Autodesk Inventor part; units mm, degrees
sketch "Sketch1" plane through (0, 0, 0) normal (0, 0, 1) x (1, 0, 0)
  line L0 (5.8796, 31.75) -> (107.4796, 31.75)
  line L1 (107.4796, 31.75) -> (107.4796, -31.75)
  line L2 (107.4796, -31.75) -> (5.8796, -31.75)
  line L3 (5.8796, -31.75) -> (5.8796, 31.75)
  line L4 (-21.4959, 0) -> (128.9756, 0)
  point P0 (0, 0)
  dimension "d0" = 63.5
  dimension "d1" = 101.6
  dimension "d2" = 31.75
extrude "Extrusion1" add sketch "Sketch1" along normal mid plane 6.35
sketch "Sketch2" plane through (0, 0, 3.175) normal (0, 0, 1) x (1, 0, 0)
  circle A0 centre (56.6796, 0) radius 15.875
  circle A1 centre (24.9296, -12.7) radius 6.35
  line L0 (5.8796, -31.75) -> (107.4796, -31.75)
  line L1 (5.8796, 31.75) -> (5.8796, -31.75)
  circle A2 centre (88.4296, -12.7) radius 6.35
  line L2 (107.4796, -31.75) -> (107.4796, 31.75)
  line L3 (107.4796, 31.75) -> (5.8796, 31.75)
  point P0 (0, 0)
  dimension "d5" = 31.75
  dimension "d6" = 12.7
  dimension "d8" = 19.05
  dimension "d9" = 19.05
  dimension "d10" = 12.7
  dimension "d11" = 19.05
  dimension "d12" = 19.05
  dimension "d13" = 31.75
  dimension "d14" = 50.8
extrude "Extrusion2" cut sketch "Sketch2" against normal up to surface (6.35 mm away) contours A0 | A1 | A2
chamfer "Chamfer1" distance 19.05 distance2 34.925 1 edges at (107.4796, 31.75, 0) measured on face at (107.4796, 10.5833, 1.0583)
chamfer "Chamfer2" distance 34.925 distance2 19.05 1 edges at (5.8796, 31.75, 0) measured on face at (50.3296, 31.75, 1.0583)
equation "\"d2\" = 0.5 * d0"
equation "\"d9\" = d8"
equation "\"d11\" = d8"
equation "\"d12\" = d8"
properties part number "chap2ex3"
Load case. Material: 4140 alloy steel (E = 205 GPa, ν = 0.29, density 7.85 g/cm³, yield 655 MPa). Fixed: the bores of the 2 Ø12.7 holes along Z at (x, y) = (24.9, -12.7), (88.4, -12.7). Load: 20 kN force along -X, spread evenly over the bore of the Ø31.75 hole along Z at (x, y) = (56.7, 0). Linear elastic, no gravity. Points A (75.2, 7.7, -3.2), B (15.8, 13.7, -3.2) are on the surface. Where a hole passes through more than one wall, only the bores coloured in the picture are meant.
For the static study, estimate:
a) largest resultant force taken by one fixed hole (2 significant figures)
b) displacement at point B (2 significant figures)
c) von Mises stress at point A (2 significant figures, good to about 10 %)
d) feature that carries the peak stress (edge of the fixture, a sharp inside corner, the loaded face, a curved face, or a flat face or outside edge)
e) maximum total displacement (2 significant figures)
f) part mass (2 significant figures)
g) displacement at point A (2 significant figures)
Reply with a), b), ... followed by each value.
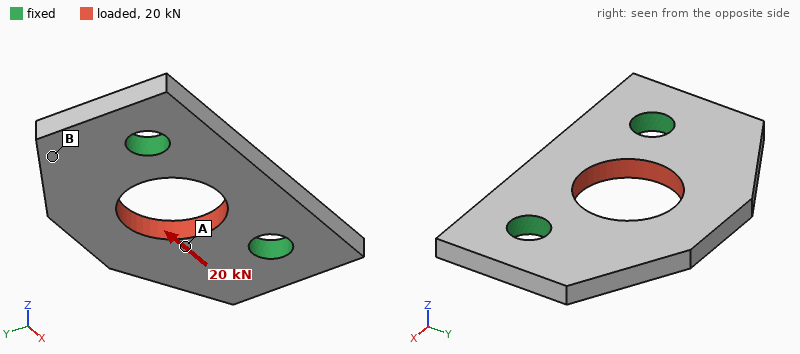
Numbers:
a) 10 kN
b) 12 µm
c) 61 MPa
d) edge of the fixture
e) 19 µm
f) 240 g
g) 13 µm
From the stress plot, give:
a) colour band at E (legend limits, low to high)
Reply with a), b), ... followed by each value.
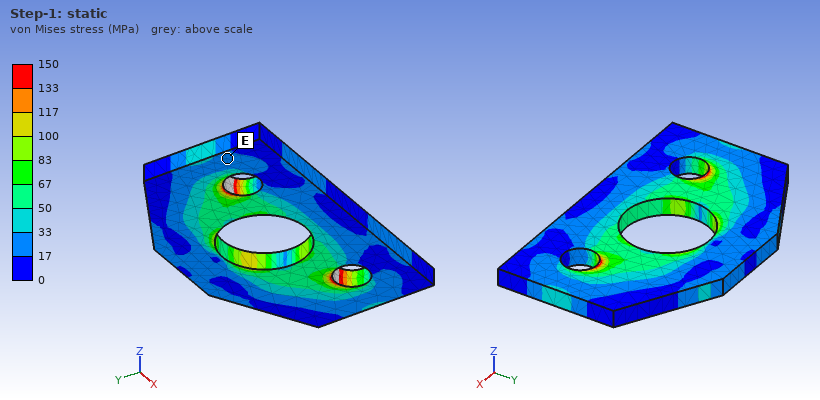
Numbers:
a) 17 to 33 MPa
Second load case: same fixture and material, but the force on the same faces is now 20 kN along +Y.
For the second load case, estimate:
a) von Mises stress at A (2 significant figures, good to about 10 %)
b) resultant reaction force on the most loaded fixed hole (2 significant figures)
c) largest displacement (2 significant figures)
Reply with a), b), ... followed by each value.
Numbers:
a) 58 MPa
b) 10 kN
c) 14 µm
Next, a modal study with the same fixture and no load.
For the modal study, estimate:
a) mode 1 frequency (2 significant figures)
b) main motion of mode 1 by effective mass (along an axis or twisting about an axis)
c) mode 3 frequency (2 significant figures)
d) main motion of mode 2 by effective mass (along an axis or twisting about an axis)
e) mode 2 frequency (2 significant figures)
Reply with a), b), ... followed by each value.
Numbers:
a) 3100 Hz
b) along Z
c) 9100 Hz
d) twisting about Y
e) 6200 Hz
